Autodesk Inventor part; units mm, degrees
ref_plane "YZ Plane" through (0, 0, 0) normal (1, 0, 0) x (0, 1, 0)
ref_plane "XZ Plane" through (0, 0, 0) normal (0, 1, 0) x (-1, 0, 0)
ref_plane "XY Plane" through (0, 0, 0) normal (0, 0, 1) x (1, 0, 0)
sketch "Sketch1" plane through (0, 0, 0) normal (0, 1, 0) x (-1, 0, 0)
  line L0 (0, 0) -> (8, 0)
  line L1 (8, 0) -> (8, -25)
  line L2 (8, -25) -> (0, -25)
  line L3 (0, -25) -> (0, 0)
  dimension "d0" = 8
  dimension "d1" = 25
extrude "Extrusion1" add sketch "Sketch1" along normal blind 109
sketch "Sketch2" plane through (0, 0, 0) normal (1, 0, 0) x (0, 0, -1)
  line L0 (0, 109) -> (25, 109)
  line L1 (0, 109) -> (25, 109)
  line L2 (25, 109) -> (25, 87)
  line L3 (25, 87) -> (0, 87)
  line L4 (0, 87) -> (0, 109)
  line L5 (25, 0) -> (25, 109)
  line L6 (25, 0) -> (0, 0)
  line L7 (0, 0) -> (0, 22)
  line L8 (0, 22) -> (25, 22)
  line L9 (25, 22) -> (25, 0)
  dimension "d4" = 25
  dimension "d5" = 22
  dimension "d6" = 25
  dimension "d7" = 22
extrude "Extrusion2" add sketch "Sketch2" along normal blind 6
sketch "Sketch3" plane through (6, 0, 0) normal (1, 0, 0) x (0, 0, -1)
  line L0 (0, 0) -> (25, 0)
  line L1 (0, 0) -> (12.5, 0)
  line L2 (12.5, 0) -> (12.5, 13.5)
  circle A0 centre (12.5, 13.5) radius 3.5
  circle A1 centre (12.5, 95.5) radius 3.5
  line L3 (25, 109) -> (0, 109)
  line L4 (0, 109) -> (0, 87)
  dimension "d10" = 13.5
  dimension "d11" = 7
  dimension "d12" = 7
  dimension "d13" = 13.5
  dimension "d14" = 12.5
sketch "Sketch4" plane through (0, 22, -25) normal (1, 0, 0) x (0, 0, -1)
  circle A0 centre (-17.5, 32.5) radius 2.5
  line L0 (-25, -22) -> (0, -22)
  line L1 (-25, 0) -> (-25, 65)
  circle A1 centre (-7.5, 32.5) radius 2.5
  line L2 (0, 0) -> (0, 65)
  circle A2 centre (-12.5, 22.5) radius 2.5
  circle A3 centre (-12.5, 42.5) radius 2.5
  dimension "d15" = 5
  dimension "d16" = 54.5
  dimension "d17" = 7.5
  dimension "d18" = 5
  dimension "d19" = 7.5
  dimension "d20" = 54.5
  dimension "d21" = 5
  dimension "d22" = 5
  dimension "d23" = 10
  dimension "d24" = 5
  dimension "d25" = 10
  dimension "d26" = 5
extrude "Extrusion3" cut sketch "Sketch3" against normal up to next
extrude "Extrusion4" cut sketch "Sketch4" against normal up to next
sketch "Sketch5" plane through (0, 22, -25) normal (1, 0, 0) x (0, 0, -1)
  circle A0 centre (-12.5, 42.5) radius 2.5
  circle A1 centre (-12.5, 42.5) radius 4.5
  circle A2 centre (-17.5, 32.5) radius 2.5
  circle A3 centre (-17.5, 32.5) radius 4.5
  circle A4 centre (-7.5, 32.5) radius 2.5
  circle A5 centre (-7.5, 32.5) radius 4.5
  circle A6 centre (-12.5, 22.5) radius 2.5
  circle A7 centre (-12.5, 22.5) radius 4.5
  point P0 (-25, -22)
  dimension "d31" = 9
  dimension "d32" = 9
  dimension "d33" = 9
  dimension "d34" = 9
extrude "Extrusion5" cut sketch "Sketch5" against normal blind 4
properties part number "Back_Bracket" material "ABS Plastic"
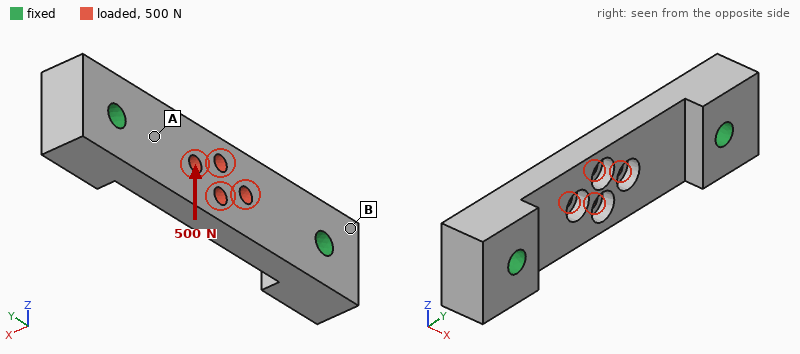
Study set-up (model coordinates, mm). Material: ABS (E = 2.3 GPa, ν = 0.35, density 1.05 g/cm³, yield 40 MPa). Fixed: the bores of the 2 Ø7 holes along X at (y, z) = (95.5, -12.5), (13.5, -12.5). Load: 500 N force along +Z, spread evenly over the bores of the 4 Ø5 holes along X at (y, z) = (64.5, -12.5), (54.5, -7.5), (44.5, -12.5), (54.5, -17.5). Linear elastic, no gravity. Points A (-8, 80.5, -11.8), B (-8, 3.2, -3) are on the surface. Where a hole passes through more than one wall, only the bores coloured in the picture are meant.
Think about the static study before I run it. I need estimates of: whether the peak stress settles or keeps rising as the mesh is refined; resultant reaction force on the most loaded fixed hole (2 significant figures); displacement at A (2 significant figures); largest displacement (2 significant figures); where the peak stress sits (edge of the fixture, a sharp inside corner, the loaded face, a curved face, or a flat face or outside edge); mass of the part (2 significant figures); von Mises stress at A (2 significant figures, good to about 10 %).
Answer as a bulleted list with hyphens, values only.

- keeps rising
- 250 N
- 0.062 mm
- 0.18 mm
- edge of the fixture
- 27 g
- 4.6 MPa
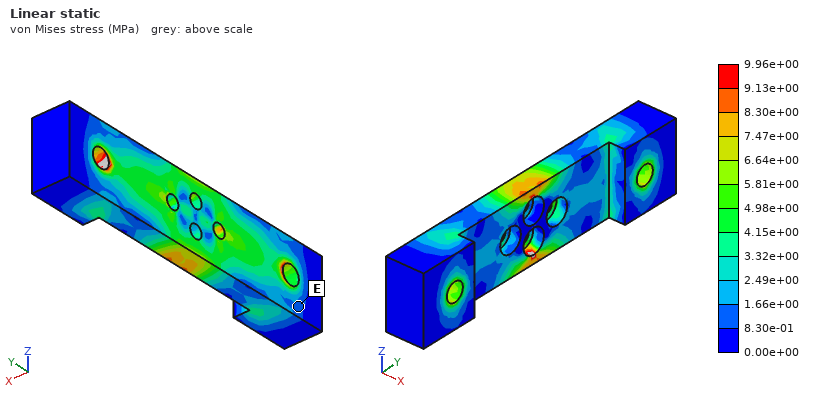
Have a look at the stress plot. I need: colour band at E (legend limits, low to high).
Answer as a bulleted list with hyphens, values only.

- 8.30e-01 to 1.66e+00 MPa
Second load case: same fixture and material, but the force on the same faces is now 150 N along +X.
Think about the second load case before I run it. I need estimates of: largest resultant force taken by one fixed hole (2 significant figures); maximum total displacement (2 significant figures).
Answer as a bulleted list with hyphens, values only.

- 92 N
- 0.17 mm
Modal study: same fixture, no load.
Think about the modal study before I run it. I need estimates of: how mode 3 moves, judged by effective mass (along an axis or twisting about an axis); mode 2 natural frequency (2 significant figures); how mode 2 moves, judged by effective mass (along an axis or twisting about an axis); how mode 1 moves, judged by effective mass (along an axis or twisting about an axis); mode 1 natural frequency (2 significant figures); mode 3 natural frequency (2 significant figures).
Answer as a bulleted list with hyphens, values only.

- twisting about Y
- 3500 Hz
- along Z
- along X
- 2200 Hz
- 3800 Hz
